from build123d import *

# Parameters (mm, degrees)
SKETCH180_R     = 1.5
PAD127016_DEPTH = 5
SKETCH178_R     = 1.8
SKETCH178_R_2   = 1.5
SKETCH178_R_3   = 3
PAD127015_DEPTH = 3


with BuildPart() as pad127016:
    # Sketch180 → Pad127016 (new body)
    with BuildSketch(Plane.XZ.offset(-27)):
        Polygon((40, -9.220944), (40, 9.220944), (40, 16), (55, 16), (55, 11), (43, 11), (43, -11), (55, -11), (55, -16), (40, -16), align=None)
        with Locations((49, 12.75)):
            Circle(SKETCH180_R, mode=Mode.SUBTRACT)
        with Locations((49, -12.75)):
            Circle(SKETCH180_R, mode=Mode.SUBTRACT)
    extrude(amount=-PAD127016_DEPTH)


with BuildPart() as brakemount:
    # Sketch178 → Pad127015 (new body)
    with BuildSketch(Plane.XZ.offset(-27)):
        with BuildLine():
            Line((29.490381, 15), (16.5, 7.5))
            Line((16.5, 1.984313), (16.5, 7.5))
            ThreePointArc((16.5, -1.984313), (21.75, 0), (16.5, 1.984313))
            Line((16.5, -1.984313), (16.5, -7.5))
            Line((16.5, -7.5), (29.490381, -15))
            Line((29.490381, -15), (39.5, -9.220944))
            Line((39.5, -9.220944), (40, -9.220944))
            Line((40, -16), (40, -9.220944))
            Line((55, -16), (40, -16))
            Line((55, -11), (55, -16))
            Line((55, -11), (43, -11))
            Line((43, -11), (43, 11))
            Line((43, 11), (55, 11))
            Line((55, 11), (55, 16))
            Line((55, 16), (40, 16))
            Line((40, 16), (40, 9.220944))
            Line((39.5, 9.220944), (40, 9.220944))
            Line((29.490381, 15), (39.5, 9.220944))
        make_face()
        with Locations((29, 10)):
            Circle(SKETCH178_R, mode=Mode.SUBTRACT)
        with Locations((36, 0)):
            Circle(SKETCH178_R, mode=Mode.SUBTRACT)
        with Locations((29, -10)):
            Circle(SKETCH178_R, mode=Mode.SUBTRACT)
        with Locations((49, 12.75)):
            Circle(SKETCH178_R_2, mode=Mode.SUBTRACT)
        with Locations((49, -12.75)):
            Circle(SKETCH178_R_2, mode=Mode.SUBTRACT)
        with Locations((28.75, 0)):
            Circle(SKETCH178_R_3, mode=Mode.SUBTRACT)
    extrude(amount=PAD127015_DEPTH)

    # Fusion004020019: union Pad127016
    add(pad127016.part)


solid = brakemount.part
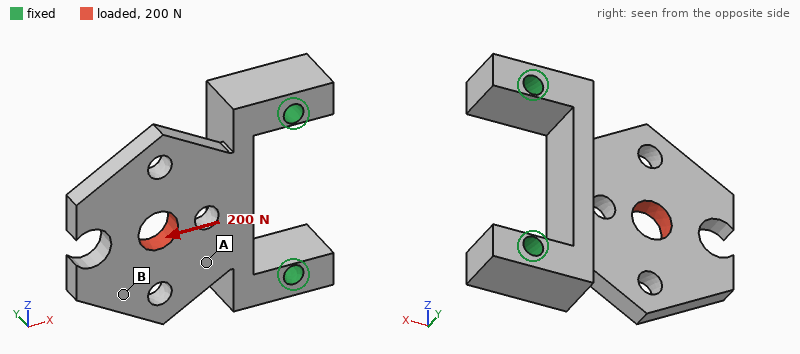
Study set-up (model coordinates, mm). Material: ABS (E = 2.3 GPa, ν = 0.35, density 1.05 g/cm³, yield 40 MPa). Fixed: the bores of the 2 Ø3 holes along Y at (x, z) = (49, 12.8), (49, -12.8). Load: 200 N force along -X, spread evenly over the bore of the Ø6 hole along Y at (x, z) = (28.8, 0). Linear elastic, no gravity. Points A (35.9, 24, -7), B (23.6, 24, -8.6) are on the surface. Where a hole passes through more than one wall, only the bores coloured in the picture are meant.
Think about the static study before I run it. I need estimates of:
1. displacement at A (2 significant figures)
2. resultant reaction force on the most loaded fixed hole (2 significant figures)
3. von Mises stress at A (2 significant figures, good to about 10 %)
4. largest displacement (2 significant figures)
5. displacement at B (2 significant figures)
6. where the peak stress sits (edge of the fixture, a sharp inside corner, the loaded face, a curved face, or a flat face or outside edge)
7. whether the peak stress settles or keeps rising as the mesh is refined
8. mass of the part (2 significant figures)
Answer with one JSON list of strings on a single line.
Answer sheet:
["0.17 mm", "110 N", "6.6 MPa", "0.42 mm", "0.32 mm", "a sharp inside corner", "keeps rising", "3.1 g"]
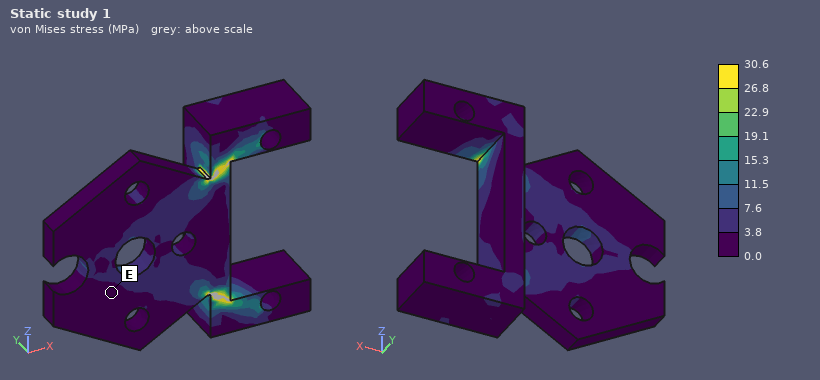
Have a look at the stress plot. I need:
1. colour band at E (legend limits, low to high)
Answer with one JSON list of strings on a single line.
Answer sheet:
["0.0 to 3.8 MPa"]
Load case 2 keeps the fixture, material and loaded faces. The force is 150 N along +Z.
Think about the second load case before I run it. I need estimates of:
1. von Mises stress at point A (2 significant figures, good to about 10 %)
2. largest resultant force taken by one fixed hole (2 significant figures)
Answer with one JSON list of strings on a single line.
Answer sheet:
["5.5 MPa", "120 N"]
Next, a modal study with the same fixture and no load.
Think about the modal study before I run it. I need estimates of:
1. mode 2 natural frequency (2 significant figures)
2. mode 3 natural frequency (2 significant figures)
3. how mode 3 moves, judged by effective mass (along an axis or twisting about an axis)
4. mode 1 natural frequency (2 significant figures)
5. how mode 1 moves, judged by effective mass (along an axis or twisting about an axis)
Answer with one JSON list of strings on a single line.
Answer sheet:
["2300 Hz", "3400 Hz", "along Z", "900 Hz", "along Y"]
